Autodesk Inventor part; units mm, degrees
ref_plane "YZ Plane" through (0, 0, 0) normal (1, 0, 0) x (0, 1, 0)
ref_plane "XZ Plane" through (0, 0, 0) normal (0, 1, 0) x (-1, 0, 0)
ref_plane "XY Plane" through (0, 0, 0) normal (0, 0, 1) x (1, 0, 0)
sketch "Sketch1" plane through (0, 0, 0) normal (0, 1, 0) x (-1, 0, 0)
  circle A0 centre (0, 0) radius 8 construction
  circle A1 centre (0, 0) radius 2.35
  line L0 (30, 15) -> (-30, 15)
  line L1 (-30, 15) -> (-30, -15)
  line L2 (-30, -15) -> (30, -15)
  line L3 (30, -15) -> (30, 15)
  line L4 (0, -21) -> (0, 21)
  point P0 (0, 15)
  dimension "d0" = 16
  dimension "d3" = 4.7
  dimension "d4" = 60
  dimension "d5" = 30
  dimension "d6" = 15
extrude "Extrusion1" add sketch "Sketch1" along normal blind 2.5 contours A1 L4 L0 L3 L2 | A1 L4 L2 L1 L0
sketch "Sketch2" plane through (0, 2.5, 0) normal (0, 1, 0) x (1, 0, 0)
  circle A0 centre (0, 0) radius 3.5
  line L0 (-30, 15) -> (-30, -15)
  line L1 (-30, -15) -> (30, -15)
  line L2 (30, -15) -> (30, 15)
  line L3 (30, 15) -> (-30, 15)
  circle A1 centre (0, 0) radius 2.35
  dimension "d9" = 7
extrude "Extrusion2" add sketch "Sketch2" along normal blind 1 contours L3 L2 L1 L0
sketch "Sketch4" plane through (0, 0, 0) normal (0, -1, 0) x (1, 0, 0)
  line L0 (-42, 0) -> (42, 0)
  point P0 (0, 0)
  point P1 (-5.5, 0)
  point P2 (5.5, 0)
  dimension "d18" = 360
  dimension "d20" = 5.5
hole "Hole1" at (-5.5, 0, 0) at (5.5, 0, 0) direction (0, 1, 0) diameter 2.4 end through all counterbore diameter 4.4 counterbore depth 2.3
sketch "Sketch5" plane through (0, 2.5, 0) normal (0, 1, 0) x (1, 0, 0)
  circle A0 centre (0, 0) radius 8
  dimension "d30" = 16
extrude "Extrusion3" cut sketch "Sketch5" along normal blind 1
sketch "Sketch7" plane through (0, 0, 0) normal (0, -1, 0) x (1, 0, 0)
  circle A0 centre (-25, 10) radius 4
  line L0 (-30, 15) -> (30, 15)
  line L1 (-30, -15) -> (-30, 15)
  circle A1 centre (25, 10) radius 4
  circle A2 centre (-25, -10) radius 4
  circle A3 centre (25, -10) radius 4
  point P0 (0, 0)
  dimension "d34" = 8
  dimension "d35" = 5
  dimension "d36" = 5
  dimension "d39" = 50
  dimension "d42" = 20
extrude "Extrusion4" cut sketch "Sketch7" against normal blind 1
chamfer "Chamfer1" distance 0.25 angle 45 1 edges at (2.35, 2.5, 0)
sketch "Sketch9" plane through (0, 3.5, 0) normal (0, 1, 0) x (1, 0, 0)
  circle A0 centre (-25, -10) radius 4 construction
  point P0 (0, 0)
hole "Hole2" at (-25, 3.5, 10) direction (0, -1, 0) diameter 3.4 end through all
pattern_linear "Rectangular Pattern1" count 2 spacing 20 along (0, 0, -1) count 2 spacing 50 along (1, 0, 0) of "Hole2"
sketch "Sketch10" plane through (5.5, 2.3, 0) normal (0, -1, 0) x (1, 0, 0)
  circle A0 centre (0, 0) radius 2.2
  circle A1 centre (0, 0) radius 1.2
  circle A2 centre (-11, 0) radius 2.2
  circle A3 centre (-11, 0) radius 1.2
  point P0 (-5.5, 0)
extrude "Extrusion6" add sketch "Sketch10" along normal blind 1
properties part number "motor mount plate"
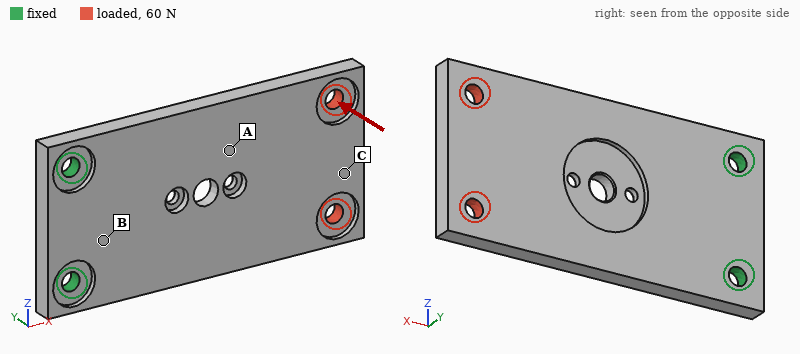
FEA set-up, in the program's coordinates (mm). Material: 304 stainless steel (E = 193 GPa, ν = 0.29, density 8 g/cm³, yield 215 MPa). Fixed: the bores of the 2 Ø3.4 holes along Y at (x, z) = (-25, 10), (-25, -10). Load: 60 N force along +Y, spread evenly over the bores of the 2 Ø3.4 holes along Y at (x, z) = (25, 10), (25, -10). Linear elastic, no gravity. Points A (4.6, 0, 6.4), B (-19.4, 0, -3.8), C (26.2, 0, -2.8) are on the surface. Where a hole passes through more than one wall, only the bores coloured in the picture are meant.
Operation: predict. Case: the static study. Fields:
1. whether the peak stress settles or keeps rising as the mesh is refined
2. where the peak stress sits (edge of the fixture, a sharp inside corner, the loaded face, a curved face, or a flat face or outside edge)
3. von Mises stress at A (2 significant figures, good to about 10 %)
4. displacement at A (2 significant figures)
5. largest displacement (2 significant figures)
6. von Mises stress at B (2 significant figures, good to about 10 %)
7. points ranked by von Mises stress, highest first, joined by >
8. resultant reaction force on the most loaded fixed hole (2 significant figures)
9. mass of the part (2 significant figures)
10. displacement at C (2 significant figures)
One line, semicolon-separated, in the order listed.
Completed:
keeps rising; edge of the fixture; 25 MPa; 0.069 mm; 0.18 mm; 43 MPa; B > A > C; 30 N; 46 g; 0.17 mm
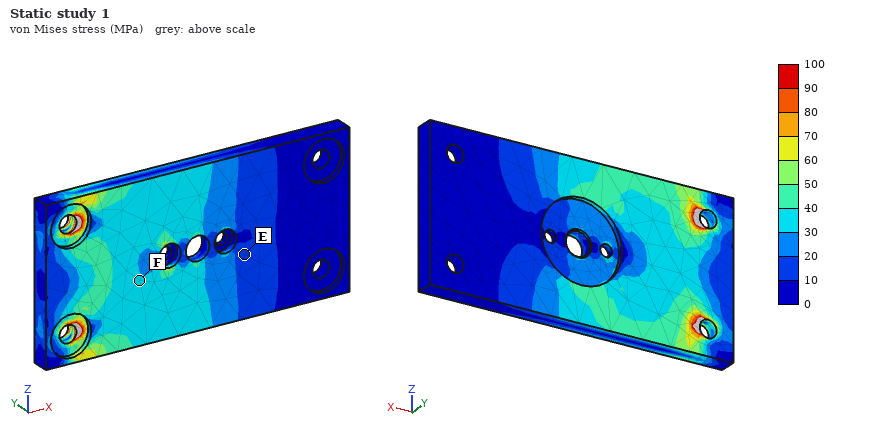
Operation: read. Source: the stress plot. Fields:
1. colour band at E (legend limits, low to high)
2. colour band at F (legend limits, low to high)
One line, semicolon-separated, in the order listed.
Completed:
10 to 20 MPa; 30 to 40 MPa
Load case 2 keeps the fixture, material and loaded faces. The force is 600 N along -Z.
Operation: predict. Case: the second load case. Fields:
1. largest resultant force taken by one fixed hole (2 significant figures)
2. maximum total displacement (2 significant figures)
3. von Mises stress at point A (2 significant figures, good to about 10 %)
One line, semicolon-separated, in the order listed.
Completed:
1.4 kN; 35 µm; 13 MPa
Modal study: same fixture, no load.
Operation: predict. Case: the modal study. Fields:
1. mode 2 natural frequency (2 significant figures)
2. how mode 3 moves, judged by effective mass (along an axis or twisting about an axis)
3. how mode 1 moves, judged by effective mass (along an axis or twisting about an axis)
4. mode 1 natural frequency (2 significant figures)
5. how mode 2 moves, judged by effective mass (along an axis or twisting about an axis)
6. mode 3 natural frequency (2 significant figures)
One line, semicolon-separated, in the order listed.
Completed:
3300 Hz; along Y; along Y; 830 Hz; twisting about X; 5100 Hz
